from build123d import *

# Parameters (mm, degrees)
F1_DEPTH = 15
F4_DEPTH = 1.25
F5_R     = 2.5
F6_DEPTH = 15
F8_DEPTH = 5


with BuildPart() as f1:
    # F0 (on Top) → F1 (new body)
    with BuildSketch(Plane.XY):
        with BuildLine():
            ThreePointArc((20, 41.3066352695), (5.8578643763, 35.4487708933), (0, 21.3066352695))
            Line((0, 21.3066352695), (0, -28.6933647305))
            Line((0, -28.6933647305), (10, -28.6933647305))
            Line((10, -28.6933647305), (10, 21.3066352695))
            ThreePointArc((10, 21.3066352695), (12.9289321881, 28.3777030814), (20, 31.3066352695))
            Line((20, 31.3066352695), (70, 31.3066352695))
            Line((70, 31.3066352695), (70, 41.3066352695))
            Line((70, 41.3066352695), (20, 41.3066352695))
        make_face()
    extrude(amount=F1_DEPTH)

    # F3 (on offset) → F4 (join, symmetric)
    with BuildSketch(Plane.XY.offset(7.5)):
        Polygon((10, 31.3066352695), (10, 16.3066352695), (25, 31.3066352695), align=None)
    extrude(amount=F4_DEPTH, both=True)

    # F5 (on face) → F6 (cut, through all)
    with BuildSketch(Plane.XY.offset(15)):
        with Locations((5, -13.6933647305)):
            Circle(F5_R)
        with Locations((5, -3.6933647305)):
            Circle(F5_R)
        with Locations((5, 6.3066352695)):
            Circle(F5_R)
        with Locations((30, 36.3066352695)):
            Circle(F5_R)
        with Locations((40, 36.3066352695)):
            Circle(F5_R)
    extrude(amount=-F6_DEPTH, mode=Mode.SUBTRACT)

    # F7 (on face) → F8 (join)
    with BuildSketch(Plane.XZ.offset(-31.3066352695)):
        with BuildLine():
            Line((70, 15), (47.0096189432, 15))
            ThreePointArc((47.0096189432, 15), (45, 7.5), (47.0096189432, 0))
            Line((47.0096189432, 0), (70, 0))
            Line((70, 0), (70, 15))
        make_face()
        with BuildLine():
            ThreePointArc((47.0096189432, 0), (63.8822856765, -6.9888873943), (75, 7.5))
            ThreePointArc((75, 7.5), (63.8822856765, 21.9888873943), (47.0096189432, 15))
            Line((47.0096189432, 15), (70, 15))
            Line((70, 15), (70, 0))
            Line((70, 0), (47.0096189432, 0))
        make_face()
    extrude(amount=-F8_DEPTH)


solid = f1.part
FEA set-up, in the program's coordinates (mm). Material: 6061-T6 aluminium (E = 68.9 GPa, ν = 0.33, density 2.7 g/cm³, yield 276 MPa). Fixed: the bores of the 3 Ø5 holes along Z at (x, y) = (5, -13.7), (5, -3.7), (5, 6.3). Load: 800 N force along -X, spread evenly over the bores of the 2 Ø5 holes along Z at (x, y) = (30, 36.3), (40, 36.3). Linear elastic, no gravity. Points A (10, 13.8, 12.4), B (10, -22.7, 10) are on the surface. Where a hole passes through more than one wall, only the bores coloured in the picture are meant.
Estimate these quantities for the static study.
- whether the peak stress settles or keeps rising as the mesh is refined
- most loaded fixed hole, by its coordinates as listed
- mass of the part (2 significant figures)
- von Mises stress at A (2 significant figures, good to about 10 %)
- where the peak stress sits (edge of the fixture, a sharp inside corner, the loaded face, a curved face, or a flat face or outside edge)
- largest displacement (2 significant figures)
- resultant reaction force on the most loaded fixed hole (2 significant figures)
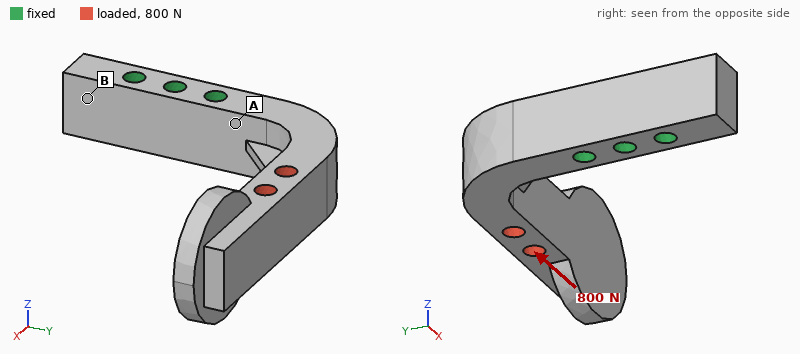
keeps rising
(5, 6.3)
51 g
69 MPa
edge of the fixture
0.30 mm
1.2 kN
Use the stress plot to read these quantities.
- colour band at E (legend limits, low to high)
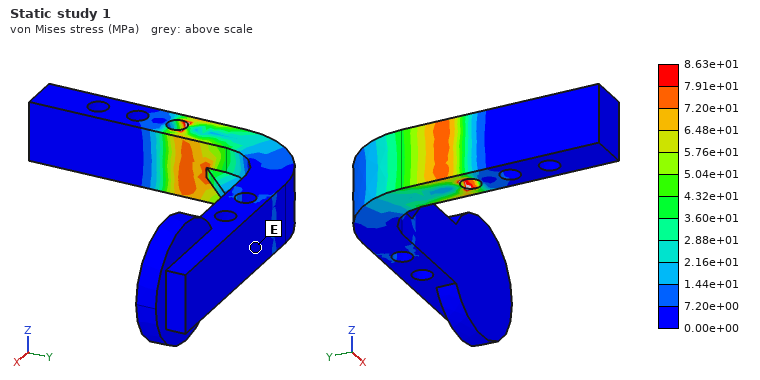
0.00e+00 to 7.20e+00 MPa
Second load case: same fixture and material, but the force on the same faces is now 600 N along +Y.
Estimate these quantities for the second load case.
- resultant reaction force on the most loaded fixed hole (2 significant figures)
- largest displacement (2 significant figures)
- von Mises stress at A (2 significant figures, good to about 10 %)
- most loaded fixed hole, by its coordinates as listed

670 N
0.43 mm
71 MPa
(5, 6.3)
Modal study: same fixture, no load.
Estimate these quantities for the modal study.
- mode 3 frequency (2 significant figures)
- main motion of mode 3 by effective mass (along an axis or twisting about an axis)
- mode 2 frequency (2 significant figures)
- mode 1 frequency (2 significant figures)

4100 Hz
along X
1100 Hz
1100 Hz
